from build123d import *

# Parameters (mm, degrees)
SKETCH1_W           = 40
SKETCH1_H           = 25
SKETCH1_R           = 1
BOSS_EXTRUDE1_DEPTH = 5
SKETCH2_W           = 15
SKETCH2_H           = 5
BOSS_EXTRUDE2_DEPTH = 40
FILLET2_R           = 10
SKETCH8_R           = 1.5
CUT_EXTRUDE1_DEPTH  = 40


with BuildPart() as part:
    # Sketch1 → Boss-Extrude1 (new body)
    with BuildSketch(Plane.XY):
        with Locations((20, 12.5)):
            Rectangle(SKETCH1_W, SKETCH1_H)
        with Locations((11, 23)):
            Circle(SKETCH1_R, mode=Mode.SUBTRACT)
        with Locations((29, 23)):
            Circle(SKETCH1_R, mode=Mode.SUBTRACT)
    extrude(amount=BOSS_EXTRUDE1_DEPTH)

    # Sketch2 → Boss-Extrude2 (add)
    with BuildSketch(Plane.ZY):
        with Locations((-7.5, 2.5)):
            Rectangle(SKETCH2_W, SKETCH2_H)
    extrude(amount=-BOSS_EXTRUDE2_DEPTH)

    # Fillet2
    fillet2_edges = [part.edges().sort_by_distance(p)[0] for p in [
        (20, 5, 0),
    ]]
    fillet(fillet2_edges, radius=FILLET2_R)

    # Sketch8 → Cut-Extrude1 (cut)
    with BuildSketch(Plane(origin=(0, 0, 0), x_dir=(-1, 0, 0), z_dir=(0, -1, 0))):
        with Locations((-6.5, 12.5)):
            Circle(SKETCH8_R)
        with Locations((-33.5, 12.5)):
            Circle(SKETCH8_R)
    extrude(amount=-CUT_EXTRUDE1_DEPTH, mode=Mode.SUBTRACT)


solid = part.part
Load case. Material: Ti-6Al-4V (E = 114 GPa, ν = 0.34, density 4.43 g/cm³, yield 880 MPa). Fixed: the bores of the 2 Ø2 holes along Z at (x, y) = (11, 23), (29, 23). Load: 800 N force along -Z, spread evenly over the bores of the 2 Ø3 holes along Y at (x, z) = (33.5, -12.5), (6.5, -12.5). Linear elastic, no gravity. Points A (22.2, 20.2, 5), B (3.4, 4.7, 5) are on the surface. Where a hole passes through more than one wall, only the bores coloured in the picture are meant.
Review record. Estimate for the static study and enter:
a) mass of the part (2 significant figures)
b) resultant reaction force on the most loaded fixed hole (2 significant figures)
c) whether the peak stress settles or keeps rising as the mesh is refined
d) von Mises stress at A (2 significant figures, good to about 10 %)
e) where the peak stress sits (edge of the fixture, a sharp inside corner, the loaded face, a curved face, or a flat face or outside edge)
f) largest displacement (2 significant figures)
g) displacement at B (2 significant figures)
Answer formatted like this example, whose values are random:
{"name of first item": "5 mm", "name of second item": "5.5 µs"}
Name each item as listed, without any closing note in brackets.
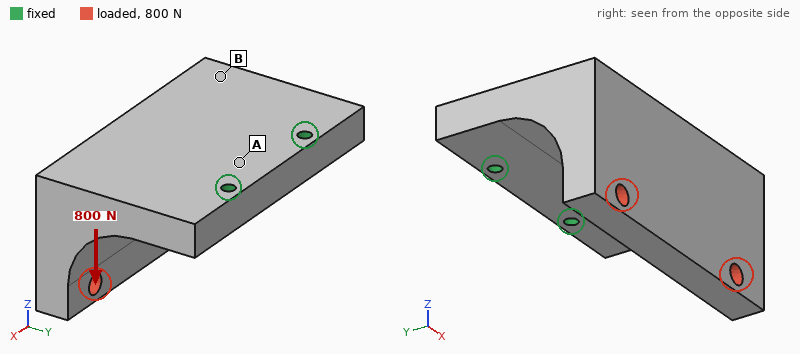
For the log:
{"mass of the part": "39 g", "resultant reaction force on the most loaded fixed hole": "400 N", "whether the peak stress settles or keeps rising as the mesh is refined": "keeps rising", "von Mises stress at A": "47 MPa", "where the peak stress sits": "edge of the fixture", "largest displacement": "0.13 mm", "displacement at B": "0.072 mm"}
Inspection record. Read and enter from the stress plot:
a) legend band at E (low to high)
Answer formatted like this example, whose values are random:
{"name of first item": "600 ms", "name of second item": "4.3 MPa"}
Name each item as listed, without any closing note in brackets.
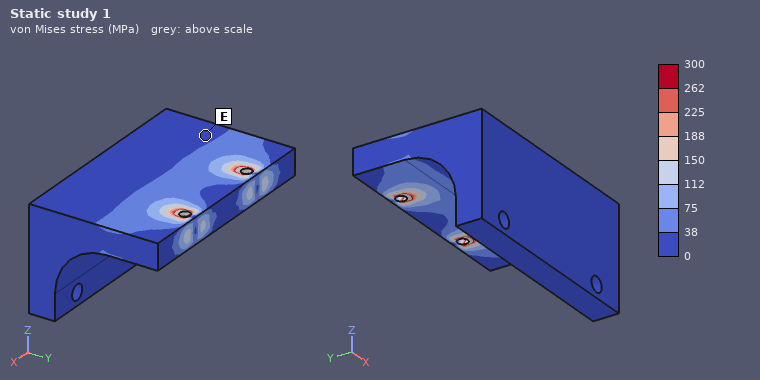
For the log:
{"legend band at E": "0 to 38 MPa"}
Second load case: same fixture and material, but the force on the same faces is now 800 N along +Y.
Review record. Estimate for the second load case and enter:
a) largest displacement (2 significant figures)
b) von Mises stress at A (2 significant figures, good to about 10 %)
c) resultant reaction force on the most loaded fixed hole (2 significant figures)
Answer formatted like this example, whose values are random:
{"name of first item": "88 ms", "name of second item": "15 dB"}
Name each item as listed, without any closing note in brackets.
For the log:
{"largest displacement": "0.13 mm", "von Mises stress at A": "42 MPa", "resultant reaction force on the most loaded fixed hole": "400 N"}
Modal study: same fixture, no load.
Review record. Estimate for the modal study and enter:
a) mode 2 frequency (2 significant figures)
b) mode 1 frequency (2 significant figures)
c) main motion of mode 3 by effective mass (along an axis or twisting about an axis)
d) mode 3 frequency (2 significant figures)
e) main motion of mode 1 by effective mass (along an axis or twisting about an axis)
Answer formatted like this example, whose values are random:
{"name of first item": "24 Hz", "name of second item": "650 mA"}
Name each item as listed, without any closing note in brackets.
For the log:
{"mode 2 frequency": "6100 Hz", "mode 1 frequency": "3000 Hz", "main motion of mode 3 by effective mass": "along X", "mode 3 frequency": "10 kHz", "main motion of mode 1 by effective mass": "along Z"}
